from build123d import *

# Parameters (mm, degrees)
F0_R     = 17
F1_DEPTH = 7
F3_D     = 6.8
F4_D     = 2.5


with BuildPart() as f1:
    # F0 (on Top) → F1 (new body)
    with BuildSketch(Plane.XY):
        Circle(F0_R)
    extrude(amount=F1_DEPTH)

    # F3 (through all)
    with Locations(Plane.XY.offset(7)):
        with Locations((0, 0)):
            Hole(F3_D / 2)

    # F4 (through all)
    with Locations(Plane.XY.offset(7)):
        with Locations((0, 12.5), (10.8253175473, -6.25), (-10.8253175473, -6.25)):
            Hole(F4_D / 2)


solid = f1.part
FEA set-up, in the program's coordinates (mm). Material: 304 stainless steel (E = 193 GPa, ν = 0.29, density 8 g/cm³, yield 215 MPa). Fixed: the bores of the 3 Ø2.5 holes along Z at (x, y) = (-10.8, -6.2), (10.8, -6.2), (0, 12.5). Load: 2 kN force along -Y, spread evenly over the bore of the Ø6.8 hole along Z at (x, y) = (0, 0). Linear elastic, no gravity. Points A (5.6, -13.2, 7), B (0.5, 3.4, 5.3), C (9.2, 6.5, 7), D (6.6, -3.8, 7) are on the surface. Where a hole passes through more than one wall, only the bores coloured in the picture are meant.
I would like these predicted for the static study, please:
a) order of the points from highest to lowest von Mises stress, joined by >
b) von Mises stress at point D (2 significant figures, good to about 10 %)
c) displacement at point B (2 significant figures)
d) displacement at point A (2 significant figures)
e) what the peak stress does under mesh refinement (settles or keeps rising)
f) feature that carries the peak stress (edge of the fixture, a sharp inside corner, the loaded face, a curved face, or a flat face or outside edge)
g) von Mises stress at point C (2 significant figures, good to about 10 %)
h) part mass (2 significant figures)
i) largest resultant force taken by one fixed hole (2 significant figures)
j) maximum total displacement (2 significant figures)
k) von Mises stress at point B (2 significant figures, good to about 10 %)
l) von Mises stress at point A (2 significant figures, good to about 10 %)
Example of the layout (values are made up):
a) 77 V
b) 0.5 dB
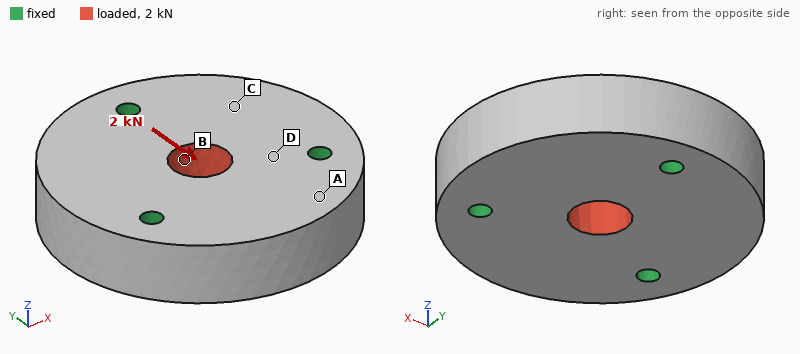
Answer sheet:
a) B > D > A > C
b) 8.5 MPa
c) 0.64 µm
d) 0.46 µm
e) keeps rising
f) edge of the fixture
g) 2.9 MPa
h) 48 g
i) 700 N
j) 0.99 µm
k) 17 MPa
l) 5.7 MPa
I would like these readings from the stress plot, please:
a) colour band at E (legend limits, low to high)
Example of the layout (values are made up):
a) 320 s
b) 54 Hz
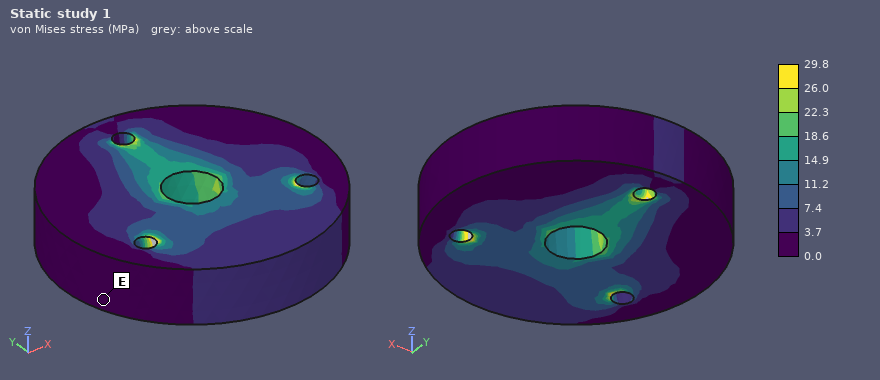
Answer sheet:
a) 0.0 to 3.7 MPa
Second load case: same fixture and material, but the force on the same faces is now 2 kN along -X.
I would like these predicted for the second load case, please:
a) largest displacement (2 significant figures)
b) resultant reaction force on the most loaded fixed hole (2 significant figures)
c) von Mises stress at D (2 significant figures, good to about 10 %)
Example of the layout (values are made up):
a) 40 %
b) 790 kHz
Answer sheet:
a) 0.94 µm
b) 680 N
c) 14 MPa
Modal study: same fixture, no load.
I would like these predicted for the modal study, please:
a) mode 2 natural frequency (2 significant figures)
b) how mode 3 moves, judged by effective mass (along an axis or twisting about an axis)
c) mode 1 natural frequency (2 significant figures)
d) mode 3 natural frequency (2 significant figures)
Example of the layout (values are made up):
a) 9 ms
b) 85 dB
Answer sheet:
a) 31 kHz
b) along Z
c) 31 kHz
d) 35 kHz
